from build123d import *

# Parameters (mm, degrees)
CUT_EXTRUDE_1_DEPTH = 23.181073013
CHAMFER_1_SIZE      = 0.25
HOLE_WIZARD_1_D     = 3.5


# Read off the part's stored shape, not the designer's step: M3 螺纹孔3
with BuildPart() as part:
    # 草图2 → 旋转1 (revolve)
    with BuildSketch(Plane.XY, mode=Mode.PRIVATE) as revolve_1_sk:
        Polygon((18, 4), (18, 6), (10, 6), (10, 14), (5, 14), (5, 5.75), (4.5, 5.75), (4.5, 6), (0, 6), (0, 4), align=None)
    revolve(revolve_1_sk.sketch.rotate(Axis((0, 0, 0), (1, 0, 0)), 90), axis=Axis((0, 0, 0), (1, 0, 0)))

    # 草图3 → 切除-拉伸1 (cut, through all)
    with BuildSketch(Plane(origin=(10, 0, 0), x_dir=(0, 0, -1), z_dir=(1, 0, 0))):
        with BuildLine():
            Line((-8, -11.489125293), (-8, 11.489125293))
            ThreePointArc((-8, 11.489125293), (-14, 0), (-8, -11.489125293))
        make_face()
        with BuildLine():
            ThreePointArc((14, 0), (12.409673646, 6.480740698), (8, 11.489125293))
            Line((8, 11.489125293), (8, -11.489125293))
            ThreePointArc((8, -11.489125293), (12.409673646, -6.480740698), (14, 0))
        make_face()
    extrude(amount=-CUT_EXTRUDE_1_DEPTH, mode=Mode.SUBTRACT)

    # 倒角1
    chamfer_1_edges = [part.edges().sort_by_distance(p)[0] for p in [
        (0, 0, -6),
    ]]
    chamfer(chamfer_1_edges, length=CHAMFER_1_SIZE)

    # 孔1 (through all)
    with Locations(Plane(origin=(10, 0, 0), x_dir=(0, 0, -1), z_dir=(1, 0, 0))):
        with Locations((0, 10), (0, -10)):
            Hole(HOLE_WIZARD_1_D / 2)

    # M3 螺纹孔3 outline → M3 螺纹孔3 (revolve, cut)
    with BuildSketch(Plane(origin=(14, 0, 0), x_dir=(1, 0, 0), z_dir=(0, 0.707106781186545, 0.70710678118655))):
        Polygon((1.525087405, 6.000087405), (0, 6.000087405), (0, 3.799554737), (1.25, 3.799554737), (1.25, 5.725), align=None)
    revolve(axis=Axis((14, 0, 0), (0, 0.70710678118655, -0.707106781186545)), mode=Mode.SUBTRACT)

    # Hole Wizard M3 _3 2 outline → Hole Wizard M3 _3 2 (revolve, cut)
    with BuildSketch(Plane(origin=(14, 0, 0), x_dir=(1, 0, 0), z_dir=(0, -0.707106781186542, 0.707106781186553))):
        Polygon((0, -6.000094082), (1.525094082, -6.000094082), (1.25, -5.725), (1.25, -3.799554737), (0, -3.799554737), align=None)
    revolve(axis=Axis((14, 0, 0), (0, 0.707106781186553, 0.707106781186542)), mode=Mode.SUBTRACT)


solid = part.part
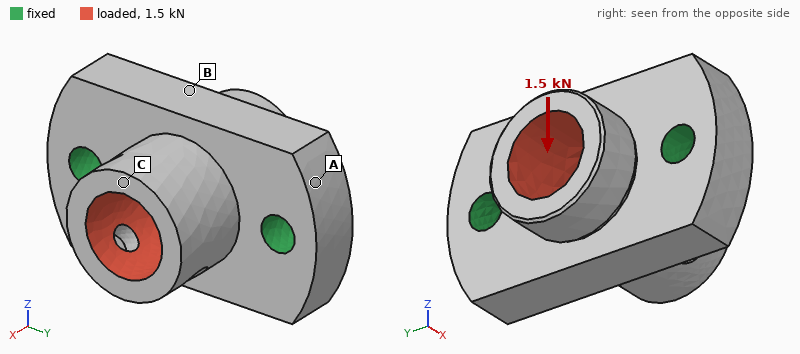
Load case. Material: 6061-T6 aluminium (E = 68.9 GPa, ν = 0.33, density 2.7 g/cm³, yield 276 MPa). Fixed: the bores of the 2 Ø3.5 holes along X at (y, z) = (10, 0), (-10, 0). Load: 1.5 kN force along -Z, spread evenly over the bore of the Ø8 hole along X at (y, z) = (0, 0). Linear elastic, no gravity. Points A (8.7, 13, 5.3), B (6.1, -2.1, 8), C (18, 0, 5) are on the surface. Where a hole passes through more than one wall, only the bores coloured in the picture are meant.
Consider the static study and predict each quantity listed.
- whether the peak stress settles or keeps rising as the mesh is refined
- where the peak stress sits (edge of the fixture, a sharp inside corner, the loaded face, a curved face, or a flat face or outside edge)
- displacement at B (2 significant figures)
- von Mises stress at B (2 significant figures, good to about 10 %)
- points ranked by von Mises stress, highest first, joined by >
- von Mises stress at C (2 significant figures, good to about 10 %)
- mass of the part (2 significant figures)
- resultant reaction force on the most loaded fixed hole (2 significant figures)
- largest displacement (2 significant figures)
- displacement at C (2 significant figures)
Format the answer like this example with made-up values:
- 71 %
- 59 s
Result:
- keeps rising
- edge of the fixture
- 4.5 µm
- 26 MPa
- B > C > A
- 13 MPa
- 6.9 g
- 750 N
- 14 µm
- 13 µm
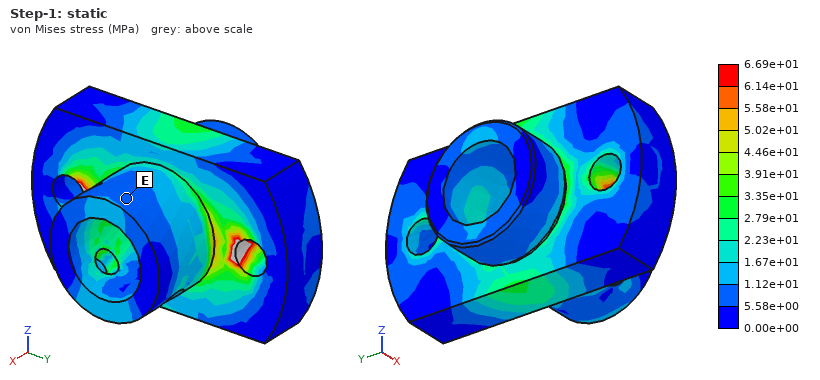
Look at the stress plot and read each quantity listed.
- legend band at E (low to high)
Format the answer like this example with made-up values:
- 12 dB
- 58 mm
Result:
- 5.58e+00 to 1.12e+01 MPa
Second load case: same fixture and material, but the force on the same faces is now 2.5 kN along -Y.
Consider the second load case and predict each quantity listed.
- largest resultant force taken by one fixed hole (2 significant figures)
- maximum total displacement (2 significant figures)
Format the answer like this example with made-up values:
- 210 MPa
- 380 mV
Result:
- 1.3 kN
- 12 µm
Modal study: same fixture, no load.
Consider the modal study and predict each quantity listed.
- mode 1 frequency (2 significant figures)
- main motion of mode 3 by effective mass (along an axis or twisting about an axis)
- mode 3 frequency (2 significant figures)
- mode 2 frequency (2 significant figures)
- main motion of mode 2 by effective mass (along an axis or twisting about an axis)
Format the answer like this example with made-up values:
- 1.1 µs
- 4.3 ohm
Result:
- 25 kHz
- along Y
- 46 kHz
- 38 kHz
- along X
